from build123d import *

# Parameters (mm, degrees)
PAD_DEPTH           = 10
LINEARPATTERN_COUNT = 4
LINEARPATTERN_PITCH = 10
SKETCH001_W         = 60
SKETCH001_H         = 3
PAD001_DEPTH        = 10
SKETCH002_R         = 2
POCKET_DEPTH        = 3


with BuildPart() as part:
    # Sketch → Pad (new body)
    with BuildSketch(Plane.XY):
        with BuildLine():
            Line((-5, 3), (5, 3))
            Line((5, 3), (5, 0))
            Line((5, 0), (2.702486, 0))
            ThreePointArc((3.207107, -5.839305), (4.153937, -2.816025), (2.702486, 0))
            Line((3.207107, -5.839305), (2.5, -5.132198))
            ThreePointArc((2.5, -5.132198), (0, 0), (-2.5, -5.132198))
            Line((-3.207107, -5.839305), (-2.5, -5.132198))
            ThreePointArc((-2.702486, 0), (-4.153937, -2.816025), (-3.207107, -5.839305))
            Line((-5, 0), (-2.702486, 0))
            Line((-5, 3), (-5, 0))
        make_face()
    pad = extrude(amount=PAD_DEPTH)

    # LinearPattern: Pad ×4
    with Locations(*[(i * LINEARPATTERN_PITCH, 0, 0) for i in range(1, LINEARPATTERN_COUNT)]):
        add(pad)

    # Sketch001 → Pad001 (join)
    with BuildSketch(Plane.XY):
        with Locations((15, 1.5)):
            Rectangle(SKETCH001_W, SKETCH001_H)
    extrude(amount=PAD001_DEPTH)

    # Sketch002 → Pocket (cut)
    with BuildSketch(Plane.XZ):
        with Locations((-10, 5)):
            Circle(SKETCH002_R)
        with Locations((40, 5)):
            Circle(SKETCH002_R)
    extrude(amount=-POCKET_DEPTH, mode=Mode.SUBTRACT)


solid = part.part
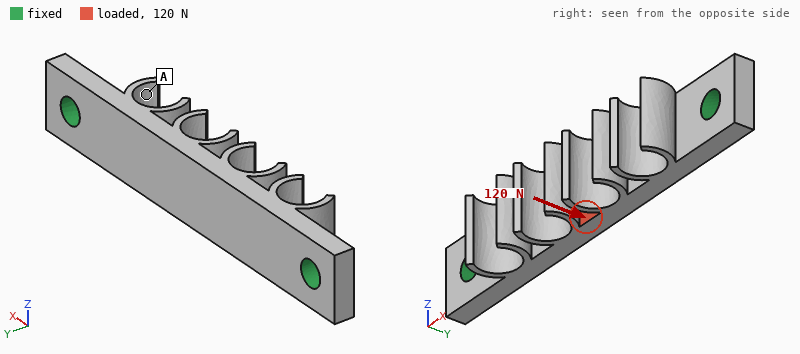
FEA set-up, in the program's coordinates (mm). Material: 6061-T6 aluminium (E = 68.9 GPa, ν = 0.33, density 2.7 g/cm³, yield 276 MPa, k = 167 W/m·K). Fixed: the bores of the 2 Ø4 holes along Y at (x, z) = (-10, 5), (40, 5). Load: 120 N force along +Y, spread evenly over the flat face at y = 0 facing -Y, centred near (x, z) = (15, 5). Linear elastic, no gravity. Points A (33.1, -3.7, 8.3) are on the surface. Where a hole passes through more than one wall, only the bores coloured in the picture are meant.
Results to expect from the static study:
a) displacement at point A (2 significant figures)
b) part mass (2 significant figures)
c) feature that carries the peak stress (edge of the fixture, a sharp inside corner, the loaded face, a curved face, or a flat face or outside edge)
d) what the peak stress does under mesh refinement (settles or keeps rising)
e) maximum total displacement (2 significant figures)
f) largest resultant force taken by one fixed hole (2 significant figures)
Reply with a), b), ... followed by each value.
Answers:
a) 13 µm
b) 6.0 g
c) edge of the fixture
d) keeps rising
e) 43 µm
f) 60 N
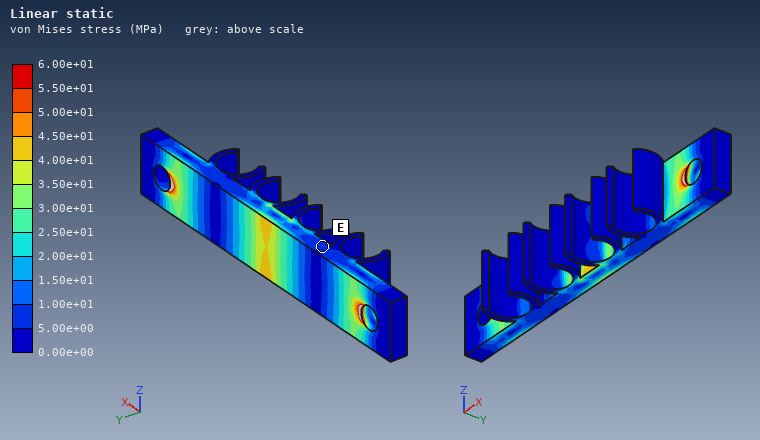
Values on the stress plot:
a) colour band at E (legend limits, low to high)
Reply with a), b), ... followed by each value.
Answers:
a) 5.00e+00 to 1.00e+01 MPa
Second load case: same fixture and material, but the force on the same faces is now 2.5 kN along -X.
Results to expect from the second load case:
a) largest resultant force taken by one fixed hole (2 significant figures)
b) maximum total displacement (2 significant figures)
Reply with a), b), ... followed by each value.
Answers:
a) 1.3 kN
b) 33 µm
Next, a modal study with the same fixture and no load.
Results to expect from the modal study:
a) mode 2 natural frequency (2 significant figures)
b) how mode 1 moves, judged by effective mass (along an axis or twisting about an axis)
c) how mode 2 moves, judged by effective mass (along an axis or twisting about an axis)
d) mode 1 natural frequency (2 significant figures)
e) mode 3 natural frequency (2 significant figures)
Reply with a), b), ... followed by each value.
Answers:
a) 11 kHz
b) along Y
c) along Z
d) 5700 Hz
e) 14 kHz
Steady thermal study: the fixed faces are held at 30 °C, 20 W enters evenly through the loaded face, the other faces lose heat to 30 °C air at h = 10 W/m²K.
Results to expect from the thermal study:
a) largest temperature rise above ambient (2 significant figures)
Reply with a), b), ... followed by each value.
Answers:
a) 46 K
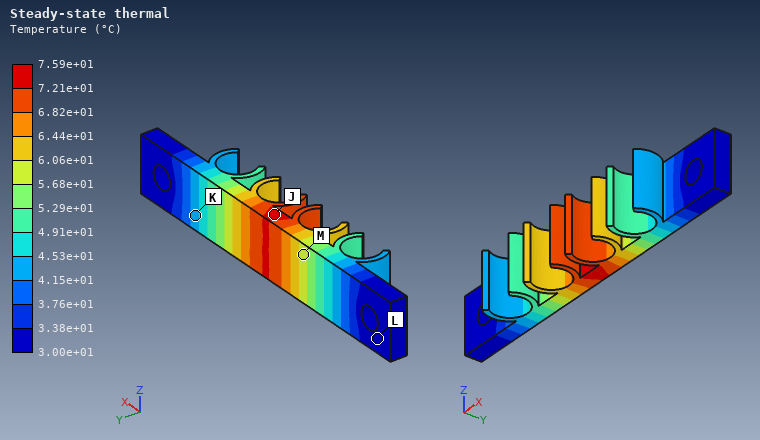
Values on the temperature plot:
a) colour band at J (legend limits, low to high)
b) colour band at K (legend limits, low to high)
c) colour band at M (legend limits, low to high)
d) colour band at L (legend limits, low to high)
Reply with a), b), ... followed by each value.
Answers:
a) 7.21e+01 to 7.59e+01 °C
b) 4.15e+01 to 4.53e+01 °C
c) 5.68e+01 to 6.06e+01 °C
d) 3.00e+01 to 3.38e+01 °C
